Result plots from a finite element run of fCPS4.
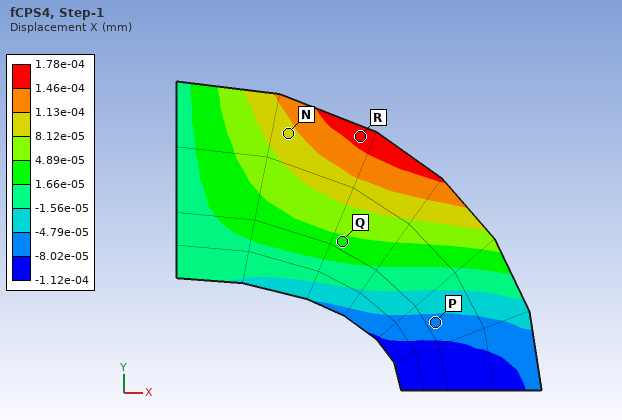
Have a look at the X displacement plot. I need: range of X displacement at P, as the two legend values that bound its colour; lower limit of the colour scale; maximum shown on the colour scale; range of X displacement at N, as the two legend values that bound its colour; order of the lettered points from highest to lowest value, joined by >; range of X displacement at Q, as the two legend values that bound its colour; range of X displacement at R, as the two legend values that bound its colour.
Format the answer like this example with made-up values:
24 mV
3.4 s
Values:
-8.02e-05 to -4.79e-05 mm
-1.12e-04 mm
1.78e-04 mm
8.12e-05 to 1.13e-04 mm
R > N > Q > P
1.66e-05 to 4.89e-05 mm
1.46e-04 to 1.78e-04 mm
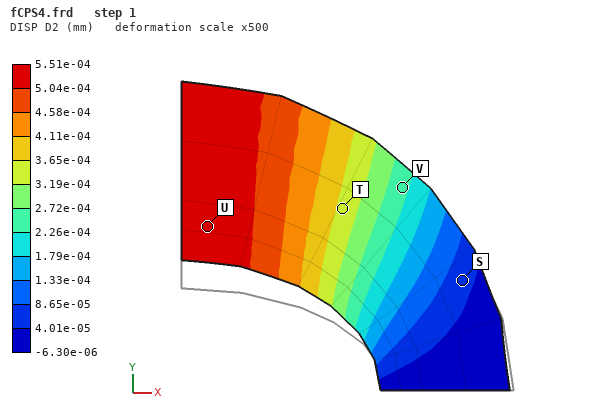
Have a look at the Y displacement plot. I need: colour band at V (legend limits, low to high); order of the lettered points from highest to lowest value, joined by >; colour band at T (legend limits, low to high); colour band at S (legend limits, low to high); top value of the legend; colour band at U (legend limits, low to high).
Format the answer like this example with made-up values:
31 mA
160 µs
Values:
2.26e-04 to 2.72e-04 mm
U > T > V > S
3.19e-04 to 3.65e-04 mm
4.01e-05 to 8.65e-05 mm
5.51e-04 mm
5.04e-04 to 5.51e-04 mm
